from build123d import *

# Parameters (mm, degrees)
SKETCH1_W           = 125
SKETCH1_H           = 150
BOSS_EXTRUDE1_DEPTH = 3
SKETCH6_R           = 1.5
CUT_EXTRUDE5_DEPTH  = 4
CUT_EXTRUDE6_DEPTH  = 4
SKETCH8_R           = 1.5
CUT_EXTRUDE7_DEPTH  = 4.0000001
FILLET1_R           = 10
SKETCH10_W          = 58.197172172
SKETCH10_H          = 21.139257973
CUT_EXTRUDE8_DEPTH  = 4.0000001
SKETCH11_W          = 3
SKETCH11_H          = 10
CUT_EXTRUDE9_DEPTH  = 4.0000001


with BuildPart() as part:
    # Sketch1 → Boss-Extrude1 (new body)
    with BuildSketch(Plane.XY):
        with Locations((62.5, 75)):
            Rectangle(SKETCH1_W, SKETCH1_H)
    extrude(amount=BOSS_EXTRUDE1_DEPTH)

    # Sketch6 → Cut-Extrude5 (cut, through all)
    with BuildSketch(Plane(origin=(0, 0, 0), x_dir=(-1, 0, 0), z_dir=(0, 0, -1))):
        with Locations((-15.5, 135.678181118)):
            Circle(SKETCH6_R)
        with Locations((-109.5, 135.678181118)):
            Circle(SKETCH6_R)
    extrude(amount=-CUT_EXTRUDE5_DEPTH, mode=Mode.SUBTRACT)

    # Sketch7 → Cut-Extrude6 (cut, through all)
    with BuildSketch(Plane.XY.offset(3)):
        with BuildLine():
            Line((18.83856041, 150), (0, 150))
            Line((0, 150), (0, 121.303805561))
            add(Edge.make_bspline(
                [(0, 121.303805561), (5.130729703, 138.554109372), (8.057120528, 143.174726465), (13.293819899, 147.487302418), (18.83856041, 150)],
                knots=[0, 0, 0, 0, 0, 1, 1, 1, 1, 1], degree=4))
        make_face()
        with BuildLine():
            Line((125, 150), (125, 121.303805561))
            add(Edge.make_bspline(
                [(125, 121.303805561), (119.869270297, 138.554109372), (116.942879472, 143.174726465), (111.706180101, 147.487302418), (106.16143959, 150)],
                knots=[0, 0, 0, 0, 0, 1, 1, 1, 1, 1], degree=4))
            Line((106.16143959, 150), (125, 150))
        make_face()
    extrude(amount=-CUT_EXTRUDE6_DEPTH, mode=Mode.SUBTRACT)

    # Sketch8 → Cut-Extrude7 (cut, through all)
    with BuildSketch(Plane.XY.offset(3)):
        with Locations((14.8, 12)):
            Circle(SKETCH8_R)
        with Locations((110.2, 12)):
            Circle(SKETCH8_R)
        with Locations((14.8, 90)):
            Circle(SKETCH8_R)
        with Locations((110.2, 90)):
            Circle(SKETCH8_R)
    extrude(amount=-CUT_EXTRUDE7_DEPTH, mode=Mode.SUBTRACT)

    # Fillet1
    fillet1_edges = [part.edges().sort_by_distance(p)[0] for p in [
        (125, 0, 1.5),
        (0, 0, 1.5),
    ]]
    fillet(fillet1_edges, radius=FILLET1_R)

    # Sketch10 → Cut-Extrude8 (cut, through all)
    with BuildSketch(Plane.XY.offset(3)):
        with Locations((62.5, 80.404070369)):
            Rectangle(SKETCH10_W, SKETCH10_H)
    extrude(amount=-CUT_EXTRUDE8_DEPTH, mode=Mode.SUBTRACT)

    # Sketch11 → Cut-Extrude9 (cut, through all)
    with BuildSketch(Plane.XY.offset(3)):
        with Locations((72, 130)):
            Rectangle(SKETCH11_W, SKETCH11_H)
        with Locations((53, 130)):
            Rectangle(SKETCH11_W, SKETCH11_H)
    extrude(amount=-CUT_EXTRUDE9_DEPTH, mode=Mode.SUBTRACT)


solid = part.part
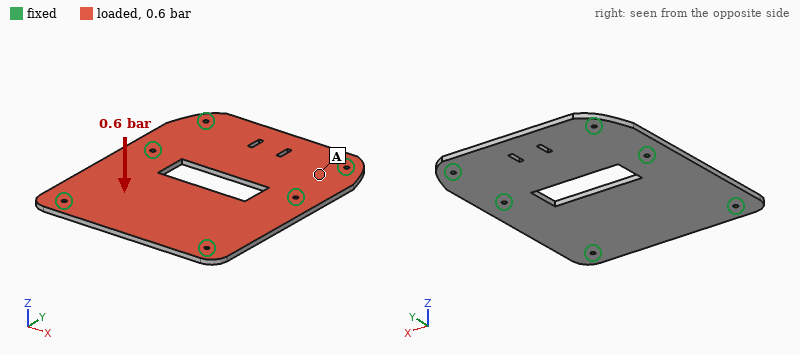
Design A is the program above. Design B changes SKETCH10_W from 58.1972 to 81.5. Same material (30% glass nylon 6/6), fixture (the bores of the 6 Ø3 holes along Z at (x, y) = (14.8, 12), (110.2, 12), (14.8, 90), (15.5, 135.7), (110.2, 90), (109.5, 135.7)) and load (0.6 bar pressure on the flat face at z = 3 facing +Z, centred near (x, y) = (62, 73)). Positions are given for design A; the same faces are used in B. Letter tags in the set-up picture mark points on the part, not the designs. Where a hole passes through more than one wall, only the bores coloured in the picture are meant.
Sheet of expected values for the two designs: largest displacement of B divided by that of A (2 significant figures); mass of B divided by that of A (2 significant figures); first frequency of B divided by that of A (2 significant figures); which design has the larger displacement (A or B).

1.3
0.97
0.89
B
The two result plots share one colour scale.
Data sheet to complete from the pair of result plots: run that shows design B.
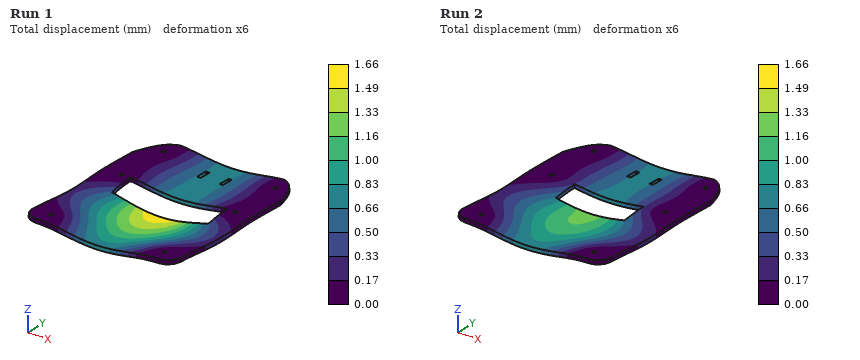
Run 1
